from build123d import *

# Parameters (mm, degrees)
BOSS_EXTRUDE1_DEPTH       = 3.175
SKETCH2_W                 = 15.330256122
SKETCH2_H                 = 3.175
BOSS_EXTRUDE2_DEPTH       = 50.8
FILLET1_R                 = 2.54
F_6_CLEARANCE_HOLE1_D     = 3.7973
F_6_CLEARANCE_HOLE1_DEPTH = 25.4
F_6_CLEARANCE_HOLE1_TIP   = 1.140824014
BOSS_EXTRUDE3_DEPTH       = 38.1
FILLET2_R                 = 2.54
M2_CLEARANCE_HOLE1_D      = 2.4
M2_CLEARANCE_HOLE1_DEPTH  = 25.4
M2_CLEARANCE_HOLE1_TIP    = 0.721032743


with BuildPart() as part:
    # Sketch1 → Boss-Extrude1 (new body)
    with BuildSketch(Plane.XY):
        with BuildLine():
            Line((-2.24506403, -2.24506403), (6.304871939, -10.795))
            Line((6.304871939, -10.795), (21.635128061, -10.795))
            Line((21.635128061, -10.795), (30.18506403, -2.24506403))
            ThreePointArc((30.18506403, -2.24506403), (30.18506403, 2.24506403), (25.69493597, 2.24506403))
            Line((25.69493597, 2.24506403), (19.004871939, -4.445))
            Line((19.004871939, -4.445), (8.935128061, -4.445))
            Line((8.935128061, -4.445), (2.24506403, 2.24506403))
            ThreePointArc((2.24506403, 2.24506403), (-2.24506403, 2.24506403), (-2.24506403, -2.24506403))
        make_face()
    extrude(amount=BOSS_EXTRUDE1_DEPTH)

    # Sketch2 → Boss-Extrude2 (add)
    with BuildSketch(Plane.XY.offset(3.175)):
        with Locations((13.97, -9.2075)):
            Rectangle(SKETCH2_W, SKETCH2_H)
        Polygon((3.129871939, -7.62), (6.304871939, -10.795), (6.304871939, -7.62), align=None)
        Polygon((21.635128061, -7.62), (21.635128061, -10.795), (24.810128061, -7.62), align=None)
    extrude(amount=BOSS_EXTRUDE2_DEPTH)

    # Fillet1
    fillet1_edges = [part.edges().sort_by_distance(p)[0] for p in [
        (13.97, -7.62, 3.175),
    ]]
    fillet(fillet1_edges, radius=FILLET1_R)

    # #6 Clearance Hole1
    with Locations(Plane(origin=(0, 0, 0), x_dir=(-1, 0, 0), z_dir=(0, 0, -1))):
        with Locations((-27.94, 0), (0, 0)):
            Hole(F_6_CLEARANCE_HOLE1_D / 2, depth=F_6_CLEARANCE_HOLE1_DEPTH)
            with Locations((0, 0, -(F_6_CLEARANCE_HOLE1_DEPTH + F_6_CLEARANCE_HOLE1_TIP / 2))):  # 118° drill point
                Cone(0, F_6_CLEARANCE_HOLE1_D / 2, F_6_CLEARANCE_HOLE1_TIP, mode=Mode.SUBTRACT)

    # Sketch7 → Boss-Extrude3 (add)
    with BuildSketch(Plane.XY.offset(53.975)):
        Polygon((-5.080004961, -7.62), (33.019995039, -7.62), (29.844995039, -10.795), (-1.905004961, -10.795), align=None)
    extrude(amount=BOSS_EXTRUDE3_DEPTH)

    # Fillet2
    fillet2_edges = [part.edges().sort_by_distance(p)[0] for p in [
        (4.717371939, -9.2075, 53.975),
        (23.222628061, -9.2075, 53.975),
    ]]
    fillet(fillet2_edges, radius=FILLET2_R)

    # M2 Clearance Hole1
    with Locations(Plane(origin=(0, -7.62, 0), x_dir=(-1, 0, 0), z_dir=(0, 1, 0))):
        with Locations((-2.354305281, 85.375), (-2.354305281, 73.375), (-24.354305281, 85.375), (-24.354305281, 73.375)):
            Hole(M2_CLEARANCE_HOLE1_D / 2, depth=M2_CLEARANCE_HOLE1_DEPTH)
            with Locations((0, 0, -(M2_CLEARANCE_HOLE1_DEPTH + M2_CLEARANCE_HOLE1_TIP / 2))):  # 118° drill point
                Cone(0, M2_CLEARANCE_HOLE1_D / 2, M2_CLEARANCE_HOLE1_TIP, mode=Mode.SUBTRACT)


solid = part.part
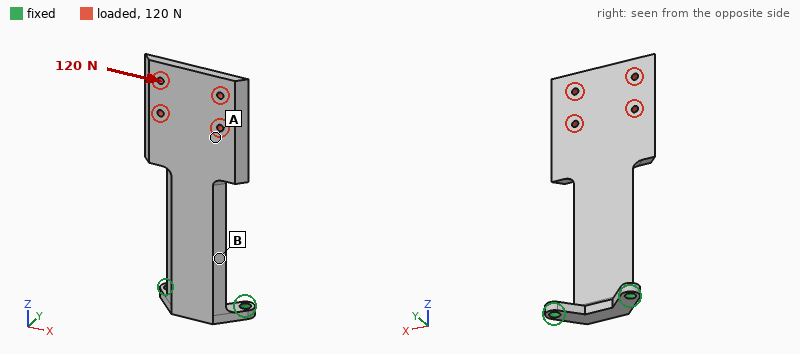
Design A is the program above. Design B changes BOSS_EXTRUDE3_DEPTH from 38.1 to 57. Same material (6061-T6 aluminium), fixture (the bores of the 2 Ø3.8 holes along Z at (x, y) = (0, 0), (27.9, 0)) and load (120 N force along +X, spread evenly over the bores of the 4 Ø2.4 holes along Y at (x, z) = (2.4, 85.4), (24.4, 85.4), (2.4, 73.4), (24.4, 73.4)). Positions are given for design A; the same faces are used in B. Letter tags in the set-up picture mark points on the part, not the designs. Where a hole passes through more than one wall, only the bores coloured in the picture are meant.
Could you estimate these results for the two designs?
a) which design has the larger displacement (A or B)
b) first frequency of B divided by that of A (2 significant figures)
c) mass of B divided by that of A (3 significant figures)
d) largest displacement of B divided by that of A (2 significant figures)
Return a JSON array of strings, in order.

["B", "0.69", "1.26", "1.2"]
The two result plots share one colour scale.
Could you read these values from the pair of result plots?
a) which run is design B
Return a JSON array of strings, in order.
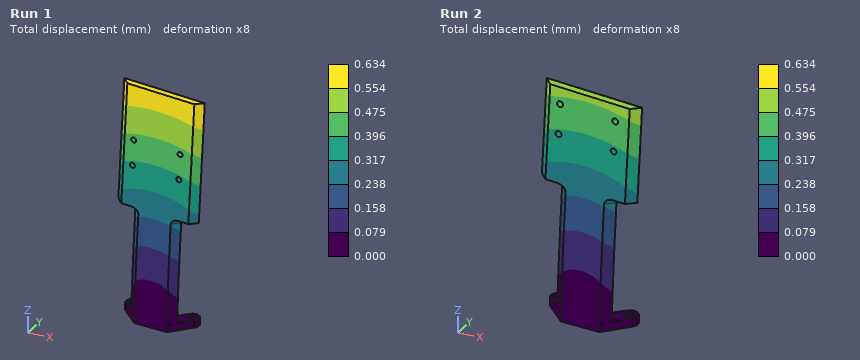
["Run 1"]
